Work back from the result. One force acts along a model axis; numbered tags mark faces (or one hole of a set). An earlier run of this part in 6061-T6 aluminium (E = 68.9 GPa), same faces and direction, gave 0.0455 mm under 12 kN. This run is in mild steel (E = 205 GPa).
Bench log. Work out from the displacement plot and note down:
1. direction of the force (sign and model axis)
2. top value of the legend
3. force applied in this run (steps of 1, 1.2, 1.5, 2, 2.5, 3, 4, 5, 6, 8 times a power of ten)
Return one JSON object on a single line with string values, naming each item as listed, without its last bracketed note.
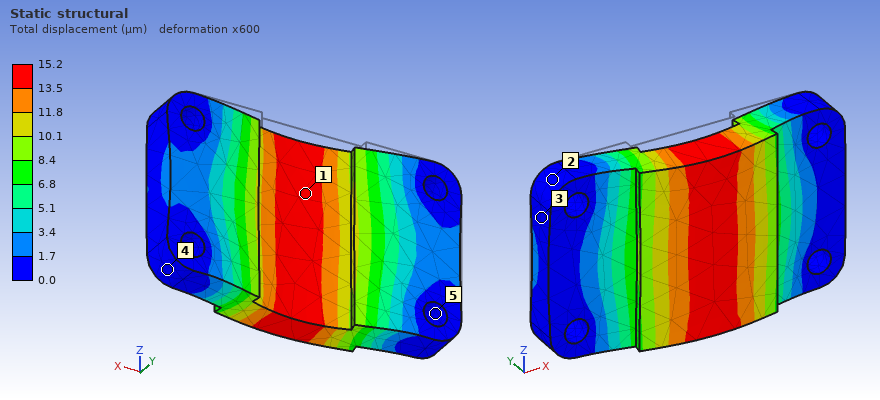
{"direction of the force": "-Y", "top value of the legend": "15.2 µm", "force applied in this run": "12 kN"}
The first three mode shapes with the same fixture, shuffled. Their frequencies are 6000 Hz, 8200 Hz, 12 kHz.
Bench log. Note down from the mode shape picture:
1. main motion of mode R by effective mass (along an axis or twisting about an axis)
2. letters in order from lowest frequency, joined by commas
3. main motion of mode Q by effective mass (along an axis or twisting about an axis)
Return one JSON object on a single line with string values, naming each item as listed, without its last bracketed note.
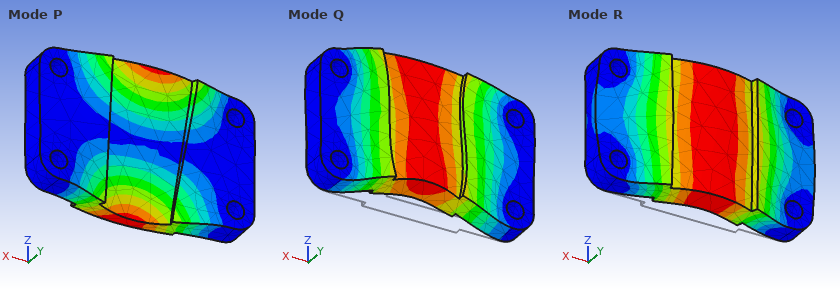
{"main motion of mode R by effective mass": "along Y", "letters in order from lowest frequency, joined by commas": "R, P, Q", "main motion of mode Q by effective mass": "along Z"}
